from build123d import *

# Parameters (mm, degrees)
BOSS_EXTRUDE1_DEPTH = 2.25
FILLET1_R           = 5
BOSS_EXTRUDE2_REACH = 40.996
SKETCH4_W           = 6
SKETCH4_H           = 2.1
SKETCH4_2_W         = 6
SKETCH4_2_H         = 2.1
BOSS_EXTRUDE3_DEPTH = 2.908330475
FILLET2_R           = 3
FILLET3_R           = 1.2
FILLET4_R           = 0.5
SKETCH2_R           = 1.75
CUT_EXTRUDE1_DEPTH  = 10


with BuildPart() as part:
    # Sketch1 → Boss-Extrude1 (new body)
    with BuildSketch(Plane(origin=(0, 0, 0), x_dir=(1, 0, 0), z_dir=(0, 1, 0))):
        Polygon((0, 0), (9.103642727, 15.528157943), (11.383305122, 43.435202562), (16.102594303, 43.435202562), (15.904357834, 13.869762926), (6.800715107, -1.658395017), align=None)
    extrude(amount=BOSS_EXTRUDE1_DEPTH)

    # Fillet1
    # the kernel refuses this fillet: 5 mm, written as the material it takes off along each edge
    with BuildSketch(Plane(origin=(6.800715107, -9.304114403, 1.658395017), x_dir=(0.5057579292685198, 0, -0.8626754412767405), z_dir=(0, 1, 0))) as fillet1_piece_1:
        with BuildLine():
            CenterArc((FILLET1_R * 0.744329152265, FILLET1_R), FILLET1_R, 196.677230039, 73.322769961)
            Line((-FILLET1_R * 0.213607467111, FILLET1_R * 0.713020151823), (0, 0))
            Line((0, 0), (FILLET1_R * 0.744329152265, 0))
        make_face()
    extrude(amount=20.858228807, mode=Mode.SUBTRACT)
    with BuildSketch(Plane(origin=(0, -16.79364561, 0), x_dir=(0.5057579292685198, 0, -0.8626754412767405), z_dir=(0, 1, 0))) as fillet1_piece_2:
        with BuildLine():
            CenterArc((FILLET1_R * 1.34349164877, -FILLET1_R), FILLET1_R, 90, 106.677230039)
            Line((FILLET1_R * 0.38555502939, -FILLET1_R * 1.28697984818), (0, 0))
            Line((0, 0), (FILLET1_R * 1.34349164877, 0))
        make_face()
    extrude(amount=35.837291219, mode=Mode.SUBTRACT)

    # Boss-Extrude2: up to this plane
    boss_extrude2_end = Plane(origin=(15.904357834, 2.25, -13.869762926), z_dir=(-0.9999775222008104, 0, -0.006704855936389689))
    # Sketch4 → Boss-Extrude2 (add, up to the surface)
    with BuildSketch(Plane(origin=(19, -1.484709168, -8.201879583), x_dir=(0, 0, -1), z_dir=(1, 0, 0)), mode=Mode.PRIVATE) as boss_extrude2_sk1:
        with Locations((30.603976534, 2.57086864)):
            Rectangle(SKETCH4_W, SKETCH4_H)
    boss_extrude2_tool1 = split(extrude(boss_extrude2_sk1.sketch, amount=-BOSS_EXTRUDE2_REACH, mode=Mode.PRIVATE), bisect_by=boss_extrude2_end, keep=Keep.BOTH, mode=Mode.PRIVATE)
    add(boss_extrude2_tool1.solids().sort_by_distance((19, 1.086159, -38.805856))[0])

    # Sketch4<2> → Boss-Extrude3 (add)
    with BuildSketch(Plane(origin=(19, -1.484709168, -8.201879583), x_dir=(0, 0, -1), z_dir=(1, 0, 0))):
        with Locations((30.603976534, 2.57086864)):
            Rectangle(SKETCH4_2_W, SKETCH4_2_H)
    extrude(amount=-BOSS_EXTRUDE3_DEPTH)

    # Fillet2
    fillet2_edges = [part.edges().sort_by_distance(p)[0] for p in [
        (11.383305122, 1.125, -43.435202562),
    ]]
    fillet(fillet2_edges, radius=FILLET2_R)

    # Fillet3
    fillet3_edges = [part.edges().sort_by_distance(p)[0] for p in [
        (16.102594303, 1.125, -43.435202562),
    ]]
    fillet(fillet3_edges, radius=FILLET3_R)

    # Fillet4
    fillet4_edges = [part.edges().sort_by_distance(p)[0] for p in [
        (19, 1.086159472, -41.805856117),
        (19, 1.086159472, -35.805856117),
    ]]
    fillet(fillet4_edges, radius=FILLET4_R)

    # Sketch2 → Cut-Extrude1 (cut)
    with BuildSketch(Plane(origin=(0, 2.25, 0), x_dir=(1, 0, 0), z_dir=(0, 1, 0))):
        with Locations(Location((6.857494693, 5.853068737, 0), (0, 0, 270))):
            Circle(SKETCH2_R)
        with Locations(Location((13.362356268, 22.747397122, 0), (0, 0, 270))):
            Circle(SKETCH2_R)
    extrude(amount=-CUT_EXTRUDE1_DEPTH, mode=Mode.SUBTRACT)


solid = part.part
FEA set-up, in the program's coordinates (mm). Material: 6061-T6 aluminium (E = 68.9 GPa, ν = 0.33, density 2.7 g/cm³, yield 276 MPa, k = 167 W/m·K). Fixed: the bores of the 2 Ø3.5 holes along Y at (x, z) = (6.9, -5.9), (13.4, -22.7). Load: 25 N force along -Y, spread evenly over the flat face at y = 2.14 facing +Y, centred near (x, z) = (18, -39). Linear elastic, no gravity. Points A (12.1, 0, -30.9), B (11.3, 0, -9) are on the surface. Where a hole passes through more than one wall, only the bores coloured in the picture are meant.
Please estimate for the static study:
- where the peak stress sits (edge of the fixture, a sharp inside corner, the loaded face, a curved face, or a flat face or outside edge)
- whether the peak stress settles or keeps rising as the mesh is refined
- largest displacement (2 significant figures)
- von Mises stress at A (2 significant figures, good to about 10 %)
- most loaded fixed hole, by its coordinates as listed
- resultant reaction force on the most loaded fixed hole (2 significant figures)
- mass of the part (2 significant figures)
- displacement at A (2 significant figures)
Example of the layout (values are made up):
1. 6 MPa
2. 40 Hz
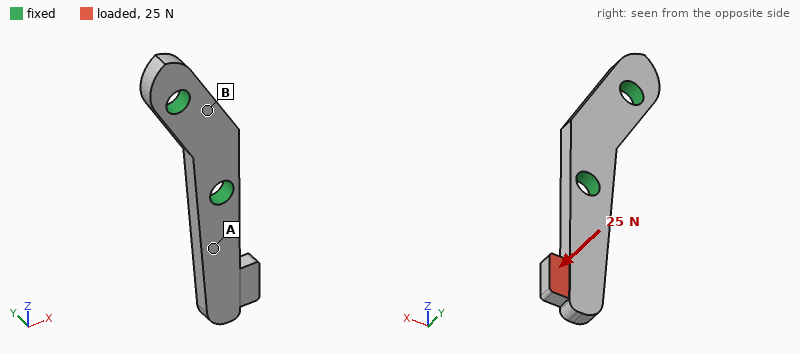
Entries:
1. edge of the fixture
2. keeps rising
3. 0.11 mm
4. 47 MPa
5. (13.4, -22.7)
6. 25 N
7. 1.6 g
8. 0.018 mm
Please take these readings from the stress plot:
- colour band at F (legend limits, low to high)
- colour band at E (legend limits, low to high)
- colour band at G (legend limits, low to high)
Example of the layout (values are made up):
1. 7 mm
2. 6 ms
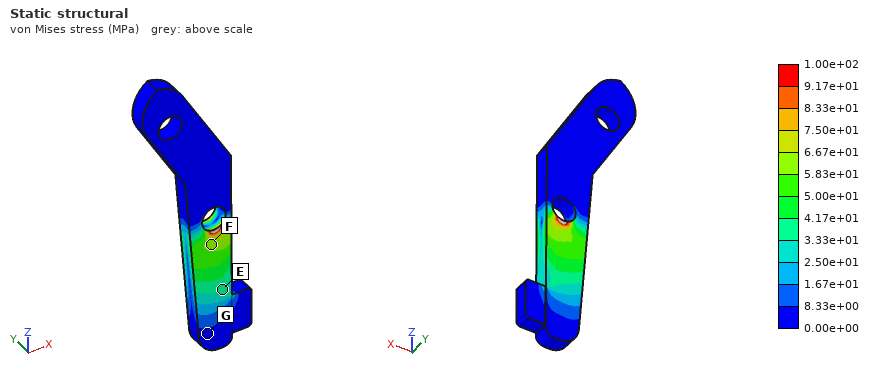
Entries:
1. 5.83e+01 to 6.67e+01 MPa
2. 3.33e+01 to 4.17e+01 MPa
3. 0.00e+00 to 8.33e+00 MPa
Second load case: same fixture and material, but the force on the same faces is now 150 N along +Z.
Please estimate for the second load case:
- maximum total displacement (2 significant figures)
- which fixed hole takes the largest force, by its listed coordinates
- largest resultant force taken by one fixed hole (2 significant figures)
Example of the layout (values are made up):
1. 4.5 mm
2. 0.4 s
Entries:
1. 90 µm
2. (13.4, -22.7)
3. 150 N
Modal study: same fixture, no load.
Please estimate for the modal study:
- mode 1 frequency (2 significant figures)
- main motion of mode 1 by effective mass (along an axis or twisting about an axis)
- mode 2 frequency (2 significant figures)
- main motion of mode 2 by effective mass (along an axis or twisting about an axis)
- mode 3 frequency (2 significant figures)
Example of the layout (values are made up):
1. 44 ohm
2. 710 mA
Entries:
1. 4700 Hz
2. along Y
3. 10 kHz
4. along X
5. 20 kHz
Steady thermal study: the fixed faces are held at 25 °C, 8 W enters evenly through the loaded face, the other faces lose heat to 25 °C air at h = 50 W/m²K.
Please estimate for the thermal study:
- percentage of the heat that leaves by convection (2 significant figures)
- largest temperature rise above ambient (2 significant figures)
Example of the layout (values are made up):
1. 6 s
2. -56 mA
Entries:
1. 6.9 %
2. 61 K
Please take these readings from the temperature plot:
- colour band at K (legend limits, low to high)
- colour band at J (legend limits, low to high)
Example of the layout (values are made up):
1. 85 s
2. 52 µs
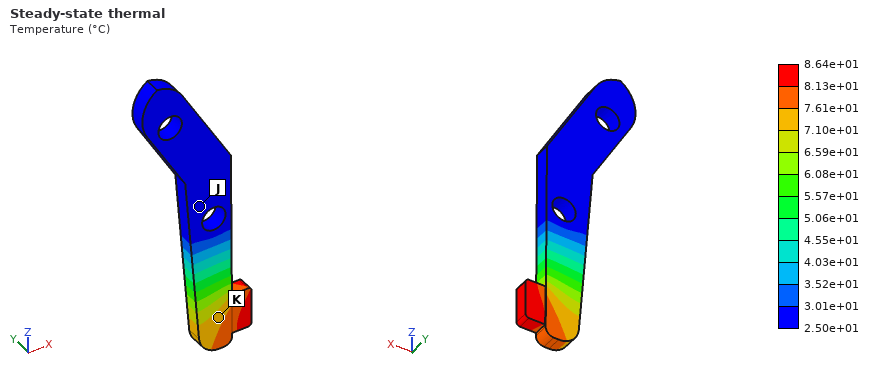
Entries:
1. 7.10e+01 to 7.61e+01 °C
2. 2.50e+01 to 3.01e+01 °C
